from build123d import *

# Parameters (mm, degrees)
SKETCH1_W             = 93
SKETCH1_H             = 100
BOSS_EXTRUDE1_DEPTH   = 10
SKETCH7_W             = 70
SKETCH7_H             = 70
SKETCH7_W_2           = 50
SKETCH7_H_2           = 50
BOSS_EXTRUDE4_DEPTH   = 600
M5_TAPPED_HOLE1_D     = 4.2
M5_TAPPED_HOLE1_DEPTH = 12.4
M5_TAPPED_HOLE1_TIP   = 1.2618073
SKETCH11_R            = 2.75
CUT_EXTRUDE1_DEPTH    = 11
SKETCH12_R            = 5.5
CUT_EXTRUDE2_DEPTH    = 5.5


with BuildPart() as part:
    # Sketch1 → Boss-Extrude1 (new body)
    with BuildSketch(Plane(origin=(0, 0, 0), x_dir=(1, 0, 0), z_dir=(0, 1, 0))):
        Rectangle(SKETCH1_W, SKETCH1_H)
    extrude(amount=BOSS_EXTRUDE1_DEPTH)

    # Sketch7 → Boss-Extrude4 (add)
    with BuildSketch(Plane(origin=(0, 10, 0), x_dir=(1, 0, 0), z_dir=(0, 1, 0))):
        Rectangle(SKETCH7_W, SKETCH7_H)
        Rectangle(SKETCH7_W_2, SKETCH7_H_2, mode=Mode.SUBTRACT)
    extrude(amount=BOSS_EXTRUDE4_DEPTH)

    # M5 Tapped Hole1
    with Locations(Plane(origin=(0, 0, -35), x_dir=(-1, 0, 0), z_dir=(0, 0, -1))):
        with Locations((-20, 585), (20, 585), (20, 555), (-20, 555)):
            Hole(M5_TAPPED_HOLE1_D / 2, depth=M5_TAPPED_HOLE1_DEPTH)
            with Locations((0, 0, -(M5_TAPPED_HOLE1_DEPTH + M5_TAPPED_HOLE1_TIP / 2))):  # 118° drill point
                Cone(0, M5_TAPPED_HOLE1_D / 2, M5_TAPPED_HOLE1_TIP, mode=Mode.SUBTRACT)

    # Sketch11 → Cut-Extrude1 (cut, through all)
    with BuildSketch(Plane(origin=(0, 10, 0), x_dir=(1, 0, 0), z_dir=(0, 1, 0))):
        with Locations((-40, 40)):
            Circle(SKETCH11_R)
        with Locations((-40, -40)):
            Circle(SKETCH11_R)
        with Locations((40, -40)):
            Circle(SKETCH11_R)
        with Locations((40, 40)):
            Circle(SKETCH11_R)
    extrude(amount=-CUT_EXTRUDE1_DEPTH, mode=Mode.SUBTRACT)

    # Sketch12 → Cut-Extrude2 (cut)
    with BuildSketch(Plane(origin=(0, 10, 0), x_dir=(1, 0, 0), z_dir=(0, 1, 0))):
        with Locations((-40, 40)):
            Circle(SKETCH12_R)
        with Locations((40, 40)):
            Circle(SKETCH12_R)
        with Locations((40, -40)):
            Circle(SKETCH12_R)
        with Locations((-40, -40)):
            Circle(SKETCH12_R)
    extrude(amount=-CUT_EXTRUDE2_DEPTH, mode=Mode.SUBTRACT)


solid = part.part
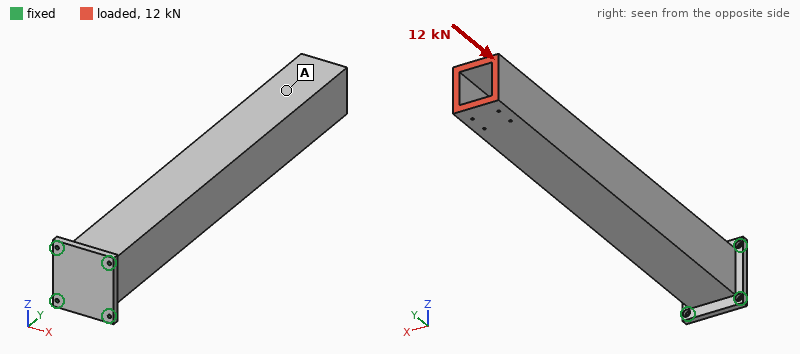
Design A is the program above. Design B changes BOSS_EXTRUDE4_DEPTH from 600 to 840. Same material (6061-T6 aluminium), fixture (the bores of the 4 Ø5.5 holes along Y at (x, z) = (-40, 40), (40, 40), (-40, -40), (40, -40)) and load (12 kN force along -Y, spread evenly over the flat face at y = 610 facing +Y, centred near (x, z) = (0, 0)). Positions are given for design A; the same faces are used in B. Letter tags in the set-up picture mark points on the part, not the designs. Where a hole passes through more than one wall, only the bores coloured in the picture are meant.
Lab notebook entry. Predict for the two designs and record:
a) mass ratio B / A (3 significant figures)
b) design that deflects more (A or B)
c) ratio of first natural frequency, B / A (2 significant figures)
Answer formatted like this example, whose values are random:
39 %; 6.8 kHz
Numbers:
1.38; B; 0.56
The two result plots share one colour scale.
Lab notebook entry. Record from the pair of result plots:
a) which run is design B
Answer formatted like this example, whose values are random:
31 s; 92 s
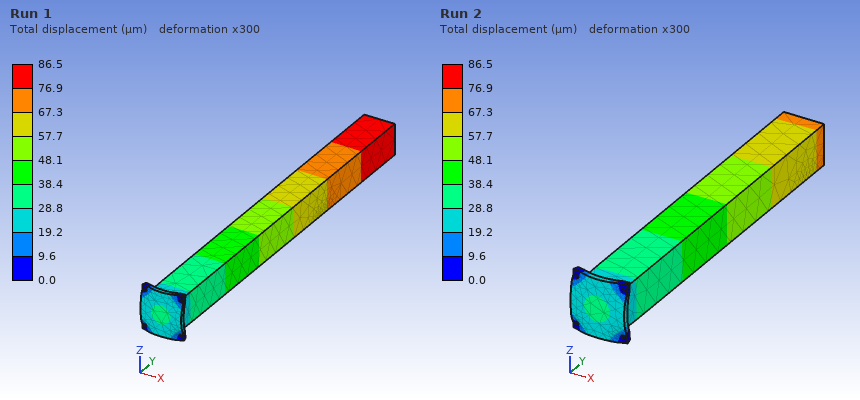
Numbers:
Run 1
